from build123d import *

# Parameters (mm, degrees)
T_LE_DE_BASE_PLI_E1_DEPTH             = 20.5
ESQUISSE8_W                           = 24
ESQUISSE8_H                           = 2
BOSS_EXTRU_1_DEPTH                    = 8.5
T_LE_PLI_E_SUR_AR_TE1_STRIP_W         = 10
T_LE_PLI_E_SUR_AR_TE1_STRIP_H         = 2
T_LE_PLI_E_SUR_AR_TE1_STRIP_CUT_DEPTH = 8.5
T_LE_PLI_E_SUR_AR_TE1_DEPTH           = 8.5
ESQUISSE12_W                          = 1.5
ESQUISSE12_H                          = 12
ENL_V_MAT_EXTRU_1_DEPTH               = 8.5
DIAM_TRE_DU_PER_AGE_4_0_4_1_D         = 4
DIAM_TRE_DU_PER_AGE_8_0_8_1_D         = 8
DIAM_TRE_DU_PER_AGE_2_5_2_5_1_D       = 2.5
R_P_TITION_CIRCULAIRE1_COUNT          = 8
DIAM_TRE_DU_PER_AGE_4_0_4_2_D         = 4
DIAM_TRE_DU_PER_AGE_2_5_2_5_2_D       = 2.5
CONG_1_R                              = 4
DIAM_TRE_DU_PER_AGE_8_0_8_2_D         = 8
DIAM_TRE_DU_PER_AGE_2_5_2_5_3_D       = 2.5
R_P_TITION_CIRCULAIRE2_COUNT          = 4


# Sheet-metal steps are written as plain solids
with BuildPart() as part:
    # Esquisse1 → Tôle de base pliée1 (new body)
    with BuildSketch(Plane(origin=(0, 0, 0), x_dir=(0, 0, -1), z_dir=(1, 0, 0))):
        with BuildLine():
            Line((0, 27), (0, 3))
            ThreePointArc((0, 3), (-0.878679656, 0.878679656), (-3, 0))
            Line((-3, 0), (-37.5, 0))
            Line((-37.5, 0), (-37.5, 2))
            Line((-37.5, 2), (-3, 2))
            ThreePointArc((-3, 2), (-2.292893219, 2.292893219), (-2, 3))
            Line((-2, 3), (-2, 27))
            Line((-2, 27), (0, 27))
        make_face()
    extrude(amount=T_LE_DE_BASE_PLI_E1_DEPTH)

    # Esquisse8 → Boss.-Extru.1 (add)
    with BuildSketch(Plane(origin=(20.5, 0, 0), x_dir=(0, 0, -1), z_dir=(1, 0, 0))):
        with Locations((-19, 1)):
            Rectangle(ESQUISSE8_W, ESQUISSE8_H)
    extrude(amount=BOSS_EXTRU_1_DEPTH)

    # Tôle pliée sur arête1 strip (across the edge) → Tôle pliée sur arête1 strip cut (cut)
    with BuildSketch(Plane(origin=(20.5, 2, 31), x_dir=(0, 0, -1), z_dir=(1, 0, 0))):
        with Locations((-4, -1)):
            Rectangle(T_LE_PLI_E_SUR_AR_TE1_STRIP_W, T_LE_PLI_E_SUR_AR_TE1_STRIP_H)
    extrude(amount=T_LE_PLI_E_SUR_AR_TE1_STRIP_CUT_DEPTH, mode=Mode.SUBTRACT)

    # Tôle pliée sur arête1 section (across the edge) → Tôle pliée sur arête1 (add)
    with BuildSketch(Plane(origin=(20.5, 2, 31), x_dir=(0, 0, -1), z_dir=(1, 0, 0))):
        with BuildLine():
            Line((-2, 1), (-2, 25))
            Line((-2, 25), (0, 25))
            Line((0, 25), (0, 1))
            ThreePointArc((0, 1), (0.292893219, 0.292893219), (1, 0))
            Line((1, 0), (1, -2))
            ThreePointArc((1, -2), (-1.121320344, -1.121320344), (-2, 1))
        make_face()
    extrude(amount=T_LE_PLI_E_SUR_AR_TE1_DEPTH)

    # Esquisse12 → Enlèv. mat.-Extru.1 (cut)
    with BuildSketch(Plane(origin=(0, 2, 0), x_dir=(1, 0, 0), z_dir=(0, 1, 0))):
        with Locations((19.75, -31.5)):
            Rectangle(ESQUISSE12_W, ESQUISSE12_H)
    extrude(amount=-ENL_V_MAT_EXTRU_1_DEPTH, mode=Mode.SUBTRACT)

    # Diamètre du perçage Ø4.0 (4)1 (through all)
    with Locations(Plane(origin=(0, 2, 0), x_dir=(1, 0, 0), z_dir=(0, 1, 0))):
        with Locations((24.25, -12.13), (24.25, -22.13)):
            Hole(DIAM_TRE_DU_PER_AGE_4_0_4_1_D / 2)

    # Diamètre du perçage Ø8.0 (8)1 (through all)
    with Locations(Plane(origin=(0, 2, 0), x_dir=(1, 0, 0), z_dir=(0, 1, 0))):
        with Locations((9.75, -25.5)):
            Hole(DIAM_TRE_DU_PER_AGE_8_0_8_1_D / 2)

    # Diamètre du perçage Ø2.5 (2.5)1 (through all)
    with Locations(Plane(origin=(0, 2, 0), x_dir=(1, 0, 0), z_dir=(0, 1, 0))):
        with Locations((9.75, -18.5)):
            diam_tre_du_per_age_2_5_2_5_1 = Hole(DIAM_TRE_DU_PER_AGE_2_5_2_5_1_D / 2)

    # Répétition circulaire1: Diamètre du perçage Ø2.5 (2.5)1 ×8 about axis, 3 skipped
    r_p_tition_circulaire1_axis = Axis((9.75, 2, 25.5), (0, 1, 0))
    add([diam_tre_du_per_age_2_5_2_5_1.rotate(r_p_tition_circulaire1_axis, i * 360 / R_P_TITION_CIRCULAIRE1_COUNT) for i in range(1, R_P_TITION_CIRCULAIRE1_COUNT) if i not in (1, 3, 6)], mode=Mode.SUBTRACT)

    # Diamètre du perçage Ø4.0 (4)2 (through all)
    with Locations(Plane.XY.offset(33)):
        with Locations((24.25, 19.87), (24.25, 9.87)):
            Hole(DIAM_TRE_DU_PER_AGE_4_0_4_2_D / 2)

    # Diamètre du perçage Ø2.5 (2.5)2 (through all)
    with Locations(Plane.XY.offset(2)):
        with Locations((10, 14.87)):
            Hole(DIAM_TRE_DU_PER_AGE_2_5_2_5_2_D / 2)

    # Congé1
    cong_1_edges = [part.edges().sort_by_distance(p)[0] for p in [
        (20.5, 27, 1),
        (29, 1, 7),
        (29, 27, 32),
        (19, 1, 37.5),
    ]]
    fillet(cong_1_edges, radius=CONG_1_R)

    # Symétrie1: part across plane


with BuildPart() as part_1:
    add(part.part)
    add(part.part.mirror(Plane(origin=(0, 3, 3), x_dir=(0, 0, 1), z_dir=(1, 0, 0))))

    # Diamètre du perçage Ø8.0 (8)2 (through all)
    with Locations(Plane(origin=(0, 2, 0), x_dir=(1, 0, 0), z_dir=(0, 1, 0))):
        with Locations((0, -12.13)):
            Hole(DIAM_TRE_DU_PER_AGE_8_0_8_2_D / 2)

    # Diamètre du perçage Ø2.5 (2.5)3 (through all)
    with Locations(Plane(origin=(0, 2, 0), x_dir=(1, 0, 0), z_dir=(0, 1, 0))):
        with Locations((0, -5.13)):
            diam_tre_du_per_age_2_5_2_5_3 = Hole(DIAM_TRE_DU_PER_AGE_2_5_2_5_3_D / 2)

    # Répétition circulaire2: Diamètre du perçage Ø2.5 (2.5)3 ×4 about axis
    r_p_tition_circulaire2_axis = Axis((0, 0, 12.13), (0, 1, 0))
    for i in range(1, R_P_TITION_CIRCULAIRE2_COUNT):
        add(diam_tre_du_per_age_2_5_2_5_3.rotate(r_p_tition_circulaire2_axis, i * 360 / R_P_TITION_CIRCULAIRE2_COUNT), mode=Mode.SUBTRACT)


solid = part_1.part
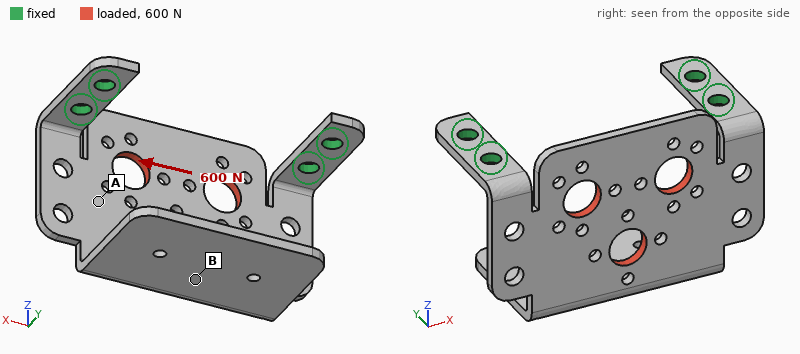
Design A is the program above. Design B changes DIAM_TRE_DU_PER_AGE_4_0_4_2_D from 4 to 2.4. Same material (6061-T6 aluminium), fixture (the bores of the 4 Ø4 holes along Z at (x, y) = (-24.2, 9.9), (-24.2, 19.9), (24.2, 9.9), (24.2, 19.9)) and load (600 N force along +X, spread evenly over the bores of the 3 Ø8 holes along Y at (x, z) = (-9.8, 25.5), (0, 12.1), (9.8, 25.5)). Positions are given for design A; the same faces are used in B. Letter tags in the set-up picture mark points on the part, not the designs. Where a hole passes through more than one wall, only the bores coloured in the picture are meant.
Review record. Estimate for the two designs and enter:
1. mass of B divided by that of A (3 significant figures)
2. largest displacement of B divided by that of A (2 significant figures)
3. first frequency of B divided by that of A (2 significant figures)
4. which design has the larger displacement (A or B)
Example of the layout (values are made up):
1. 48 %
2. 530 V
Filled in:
1. 1.01
2. 1.2
3. 0.98
4. B
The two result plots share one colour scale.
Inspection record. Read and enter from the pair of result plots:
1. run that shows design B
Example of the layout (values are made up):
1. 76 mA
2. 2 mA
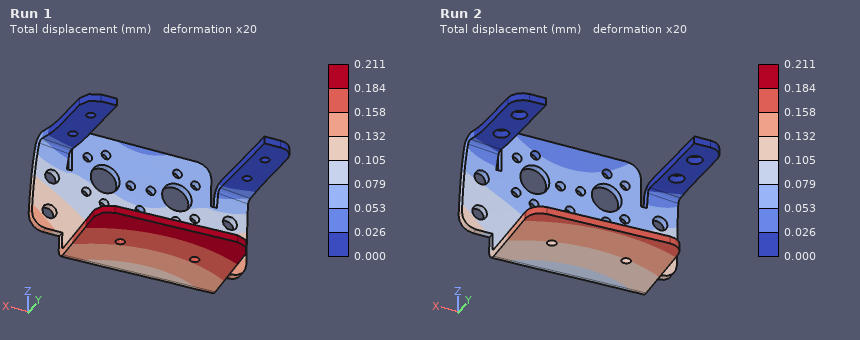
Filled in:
1. Run 1
